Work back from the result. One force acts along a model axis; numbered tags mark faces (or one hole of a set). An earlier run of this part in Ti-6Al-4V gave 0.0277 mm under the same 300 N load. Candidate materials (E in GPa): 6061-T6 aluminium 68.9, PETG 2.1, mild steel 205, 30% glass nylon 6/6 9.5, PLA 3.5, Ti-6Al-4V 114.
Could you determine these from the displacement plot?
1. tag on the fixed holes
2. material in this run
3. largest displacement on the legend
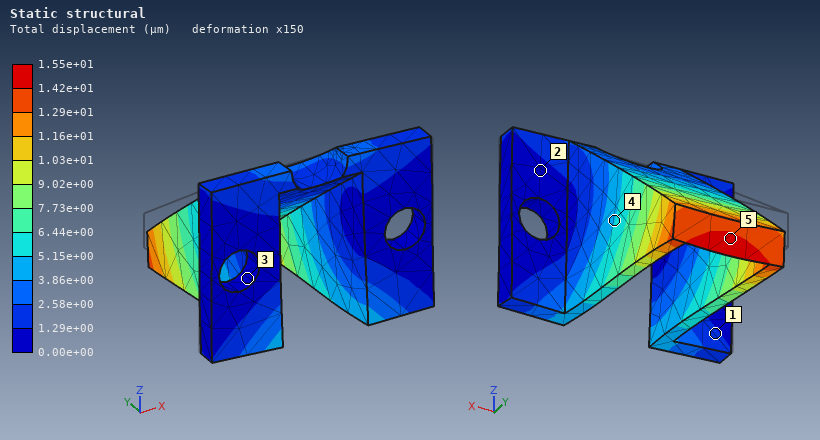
3
mild steel
1.55e+01 µm
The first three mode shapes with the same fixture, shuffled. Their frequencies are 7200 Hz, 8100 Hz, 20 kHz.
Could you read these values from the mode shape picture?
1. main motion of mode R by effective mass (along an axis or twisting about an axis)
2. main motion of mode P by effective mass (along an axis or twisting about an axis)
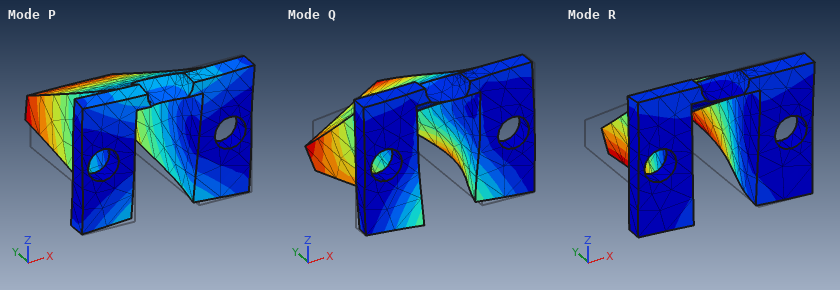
along X
along Z
